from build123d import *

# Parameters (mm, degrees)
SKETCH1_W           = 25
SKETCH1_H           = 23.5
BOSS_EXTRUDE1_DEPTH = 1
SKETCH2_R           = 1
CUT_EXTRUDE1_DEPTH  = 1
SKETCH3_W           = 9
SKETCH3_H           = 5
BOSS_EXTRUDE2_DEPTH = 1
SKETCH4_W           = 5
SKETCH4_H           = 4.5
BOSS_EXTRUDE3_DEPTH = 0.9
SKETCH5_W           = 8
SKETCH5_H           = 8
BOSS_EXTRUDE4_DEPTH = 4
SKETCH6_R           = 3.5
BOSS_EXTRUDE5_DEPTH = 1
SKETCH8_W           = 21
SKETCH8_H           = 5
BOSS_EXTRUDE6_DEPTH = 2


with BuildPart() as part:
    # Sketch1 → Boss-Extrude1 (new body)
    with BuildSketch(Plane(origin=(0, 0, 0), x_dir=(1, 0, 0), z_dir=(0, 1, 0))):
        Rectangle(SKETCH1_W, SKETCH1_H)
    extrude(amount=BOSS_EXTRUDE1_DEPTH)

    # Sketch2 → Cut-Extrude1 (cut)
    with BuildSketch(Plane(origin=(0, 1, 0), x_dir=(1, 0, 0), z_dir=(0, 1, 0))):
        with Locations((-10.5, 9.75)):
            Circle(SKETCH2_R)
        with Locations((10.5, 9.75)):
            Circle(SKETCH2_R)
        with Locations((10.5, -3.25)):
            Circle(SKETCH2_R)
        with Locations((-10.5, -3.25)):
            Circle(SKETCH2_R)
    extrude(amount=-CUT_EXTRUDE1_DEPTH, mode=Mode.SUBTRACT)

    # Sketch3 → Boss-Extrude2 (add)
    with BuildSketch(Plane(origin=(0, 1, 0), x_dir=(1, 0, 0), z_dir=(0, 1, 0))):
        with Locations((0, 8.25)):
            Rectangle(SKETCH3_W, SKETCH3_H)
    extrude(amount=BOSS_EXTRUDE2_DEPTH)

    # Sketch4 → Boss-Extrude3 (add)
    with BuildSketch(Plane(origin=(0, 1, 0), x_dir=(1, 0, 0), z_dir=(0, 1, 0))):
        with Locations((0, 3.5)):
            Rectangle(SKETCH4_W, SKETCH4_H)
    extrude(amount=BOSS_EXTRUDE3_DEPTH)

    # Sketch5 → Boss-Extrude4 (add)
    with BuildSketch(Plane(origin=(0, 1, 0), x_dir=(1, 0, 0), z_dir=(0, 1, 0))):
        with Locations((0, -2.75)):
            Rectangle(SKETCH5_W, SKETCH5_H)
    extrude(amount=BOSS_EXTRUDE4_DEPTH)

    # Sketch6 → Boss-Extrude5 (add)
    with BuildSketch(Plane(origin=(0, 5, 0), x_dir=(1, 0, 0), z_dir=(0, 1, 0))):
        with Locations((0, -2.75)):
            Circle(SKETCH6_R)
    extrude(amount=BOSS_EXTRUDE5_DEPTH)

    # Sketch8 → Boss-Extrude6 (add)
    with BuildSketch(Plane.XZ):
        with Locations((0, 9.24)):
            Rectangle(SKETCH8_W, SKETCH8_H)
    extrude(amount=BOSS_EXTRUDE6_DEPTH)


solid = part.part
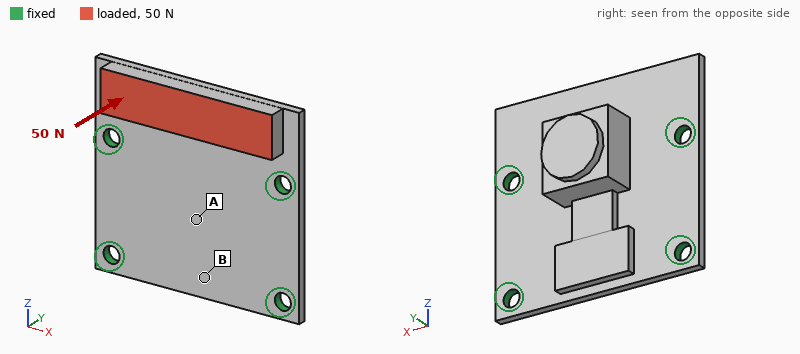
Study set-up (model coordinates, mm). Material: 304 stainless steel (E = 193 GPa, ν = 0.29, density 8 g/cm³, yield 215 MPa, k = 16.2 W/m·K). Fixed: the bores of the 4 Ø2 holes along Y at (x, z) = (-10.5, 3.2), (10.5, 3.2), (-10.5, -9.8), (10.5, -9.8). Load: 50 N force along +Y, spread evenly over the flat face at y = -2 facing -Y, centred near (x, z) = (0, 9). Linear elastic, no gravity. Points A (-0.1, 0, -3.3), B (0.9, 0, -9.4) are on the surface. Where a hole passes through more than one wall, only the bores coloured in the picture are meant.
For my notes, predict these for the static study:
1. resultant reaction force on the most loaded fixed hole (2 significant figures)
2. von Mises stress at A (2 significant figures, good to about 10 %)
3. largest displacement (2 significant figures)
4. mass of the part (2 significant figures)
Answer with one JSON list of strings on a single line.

["31 N", "11 MPa", "10.0 µm", "9.2 g"]
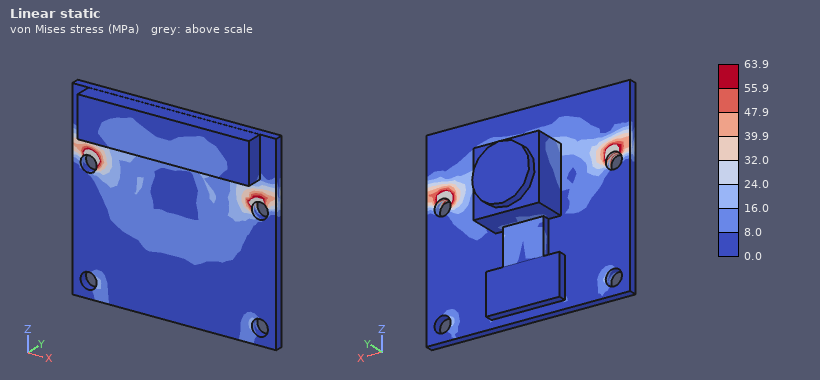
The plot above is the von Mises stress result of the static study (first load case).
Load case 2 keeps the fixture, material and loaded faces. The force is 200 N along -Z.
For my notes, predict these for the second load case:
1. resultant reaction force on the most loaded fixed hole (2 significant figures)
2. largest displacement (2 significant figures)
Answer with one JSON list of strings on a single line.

["80 N", "20 µm"]
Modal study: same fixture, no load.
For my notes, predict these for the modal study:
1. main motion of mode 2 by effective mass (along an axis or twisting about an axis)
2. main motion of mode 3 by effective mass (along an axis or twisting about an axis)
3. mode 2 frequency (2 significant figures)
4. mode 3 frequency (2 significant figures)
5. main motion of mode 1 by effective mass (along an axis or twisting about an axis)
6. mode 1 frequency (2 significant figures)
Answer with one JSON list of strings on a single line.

["along Y", "twisting about Z", "11 kHz", "19 kHz", "along Y", "7500 Hz"]
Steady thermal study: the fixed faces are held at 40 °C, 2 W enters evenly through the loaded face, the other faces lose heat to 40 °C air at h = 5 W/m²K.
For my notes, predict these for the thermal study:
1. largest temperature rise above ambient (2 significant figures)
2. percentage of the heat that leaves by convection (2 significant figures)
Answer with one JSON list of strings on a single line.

["34 K", "5.1 %"]
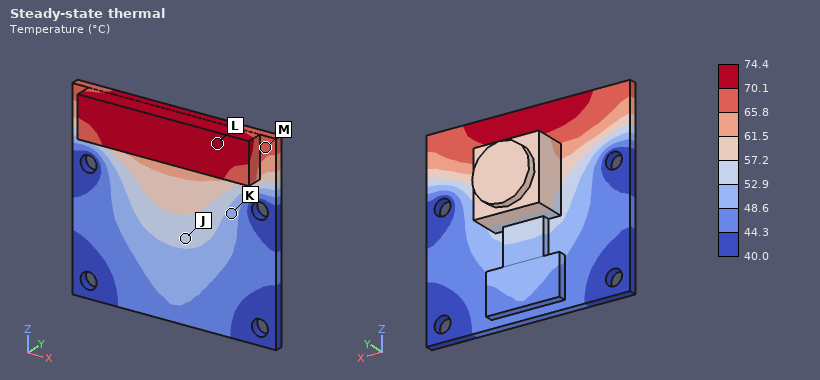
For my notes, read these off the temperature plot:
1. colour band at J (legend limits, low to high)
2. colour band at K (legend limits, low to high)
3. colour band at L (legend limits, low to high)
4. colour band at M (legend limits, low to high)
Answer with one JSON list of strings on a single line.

["52.9 to 57.2 °C", "48.6 to 52.9 °C", "70.1 to 74.4 °C", "65.8 to 70.1 °C"]
